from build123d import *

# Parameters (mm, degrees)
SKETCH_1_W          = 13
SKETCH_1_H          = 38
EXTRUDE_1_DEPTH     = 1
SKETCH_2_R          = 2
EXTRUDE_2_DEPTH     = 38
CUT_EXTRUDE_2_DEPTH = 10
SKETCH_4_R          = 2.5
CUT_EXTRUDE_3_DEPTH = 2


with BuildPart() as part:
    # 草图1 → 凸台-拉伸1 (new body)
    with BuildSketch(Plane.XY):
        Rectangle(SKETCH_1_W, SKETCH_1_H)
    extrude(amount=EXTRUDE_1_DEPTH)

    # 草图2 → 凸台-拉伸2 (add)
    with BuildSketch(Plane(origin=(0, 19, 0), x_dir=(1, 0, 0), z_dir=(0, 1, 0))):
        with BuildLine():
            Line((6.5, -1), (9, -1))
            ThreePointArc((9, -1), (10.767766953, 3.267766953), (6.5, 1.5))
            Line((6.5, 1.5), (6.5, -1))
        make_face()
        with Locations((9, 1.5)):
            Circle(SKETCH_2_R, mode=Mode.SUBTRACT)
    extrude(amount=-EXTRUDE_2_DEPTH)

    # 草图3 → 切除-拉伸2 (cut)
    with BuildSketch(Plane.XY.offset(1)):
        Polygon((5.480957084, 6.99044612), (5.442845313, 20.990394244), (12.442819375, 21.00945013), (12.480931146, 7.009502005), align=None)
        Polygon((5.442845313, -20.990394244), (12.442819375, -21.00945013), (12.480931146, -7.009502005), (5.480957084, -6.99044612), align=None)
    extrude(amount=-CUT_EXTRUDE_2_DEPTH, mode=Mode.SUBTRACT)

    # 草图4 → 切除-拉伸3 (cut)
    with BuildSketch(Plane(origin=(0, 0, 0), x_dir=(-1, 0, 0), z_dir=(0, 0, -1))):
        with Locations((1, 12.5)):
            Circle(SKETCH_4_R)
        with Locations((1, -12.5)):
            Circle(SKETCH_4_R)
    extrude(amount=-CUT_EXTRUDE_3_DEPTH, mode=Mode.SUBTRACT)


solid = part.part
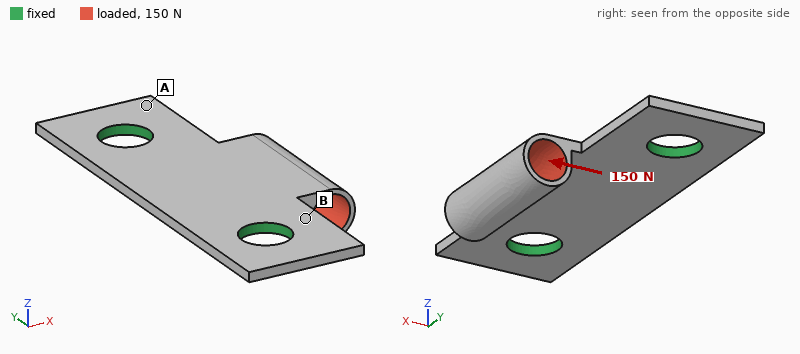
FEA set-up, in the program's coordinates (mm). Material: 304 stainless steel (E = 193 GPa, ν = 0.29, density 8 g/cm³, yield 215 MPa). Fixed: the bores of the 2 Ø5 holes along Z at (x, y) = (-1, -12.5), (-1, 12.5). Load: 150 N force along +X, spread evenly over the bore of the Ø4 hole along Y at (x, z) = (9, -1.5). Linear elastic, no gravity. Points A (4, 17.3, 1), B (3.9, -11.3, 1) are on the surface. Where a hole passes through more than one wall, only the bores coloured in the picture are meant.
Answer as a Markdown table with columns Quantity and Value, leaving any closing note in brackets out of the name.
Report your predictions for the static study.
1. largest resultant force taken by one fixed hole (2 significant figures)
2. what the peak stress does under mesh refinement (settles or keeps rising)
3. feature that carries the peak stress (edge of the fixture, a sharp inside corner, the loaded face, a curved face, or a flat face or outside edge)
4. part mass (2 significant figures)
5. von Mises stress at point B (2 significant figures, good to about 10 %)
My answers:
| Quantity | Value |
|---|---|
| largest resultant force taken by one fixed hole | 79 N |
| what the peak stress does under mesh refinement | keeps rising |
| feature that carries the peak stress | a sharp inside corner |
| part mass | 4.4 g |
| von Mises stress at point B | 56 MPa |
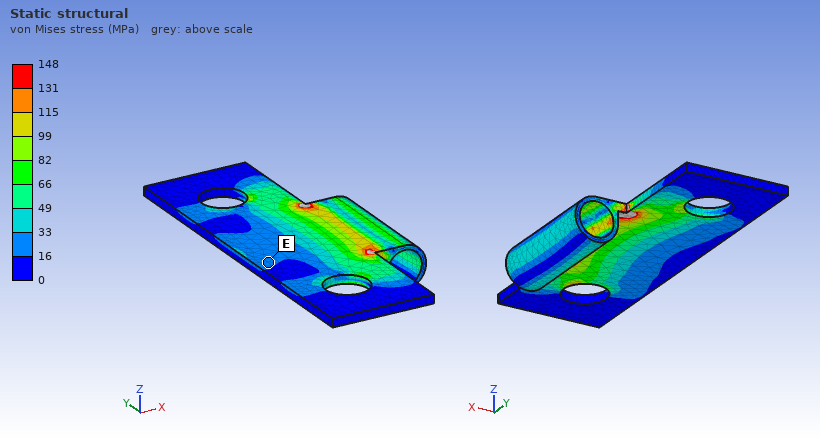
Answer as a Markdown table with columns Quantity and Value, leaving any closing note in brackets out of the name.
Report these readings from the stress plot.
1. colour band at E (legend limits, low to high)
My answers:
| Quantity | Value |
|---|---|
| colour band at E | 16 to 33 MPa |
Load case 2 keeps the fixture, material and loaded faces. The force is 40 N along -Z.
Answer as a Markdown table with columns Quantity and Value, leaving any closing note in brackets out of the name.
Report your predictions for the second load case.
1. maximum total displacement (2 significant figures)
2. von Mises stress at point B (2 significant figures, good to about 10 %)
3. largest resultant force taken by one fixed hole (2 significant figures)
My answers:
| Quantity | Value |
|---|---|
| maximum total displacement | 60 µm |
| von Mises stress at point B | 74 MPa |
| largest resultant force taken by one fixed hole | 20 N |
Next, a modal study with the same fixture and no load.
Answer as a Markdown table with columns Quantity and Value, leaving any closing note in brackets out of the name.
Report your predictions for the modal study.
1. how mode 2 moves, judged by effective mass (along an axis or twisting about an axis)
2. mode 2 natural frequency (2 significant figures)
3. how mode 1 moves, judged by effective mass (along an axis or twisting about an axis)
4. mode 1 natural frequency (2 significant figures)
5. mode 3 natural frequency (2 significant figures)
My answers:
| Quantity | Value |
|---|---|
| how mode 2 moves, judged by effective mass | along Z |
| mode 2 natural frequency | 11 kHz |
| how mode 1 moves, judged by effective mass | along Z |
| mode 1 natural frequency | 4600 Hz |
| mode 3 natural frequency | 14 kHz |
